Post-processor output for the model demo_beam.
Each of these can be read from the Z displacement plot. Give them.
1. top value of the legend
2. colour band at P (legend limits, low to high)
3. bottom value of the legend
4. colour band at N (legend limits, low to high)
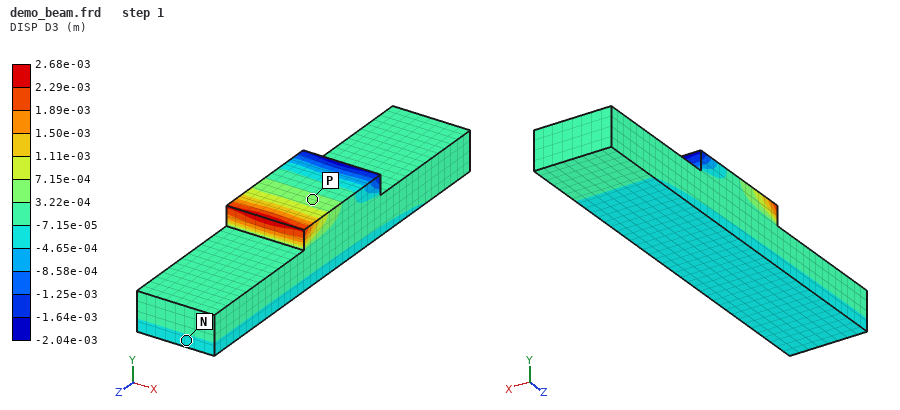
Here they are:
2.68e-03 m
3.22e-04 to 7.15e-04 m
-2.04e-03 m
-4.65e-04 to -7.15e-05 m
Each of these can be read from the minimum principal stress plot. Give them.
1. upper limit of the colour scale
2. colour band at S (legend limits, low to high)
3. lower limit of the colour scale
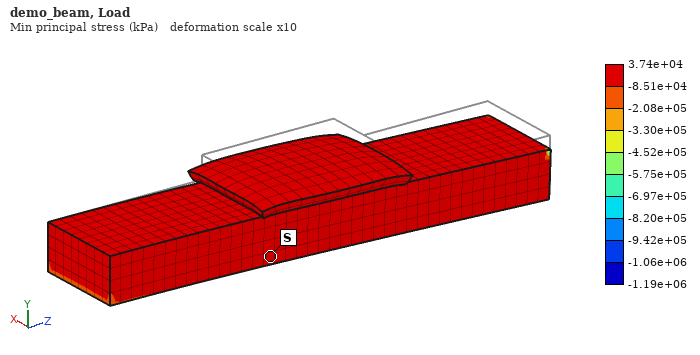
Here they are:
3.74e+04 kPa
-8.51e+04 to 3.74e+04 kPa
-1.19e+06 kPa
